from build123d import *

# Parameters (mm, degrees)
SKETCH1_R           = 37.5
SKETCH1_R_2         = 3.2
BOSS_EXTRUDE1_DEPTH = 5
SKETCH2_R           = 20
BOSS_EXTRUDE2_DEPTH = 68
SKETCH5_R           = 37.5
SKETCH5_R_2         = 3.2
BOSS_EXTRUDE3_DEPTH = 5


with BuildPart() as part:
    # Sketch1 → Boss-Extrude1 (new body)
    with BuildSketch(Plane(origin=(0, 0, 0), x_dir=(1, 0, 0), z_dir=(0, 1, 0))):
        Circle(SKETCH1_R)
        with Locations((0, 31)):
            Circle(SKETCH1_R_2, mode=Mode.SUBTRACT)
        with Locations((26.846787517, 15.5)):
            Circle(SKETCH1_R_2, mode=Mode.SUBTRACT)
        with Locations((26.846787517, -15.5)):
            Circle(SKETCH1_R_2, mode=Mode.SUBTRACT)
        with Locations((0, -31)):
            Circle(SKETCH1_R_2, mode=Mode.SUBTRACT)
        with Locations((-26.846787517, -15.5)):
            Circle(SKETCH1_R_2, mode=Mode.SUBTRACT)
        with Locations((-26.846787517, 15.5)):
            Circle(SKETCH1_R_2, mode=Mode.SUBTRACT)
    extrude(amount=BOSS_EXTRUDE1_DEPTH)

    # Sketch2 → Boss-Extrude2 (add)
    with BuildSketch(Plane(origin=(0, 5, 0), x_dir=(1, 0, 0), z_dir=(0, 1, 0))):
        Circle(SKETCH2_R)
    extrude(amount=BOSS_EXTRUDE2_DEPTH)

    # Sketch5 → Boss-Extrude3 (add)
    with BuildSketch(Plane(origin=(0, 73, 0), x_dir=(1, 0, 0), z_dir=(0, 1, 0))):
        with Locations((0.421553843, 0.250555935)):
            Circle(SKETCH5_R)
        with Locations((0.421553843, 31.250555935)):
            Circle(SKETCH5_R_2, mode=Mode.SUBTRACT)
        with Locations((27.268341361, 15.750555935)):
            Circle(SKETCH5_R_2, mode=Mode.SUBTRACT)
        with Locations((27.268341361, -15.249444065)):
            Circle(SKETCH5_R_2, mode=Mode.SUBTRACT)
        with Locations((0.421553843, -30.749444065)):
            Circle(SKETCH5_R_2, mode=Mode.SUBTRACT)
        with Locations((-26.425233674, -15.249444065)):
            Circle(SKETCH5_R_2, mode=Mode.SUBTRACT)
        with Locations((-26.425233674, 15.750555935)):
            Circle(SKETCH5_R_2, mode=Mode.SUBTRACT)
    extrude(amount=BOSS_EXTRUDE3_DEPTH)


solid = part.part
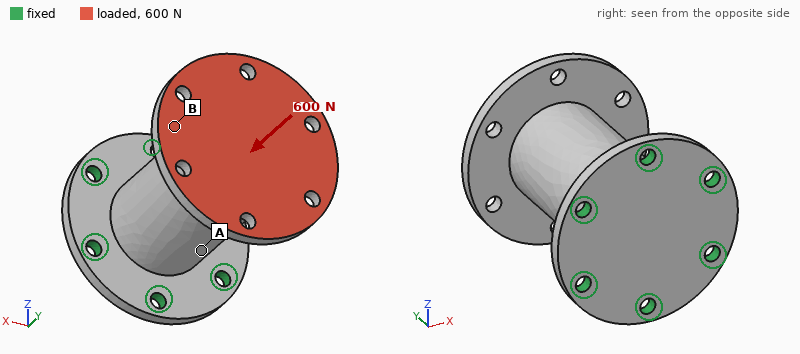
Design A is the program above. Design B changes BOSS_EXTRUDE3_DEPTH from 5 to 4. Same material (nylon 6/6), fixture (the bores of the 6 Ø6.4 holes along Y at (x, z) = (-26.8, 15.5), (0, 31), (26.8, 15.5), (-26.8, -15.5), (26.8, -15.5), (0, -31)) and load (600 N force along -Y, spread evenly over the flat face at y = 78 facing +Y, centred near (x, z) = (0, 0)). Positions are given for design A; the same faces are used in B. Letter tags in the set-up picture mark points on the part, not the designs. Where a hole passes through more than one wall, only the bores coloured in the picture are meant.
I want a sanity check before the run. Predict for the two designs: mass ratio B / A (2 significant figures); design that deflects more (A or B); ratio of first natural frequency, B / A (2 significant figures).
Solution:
0.97
B
1.1
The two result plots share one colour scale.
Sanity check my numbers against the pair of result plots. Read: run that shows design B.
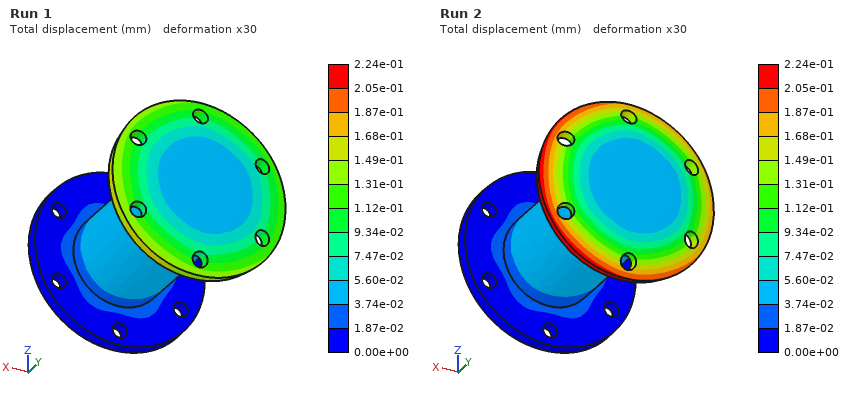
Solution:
Run 2
